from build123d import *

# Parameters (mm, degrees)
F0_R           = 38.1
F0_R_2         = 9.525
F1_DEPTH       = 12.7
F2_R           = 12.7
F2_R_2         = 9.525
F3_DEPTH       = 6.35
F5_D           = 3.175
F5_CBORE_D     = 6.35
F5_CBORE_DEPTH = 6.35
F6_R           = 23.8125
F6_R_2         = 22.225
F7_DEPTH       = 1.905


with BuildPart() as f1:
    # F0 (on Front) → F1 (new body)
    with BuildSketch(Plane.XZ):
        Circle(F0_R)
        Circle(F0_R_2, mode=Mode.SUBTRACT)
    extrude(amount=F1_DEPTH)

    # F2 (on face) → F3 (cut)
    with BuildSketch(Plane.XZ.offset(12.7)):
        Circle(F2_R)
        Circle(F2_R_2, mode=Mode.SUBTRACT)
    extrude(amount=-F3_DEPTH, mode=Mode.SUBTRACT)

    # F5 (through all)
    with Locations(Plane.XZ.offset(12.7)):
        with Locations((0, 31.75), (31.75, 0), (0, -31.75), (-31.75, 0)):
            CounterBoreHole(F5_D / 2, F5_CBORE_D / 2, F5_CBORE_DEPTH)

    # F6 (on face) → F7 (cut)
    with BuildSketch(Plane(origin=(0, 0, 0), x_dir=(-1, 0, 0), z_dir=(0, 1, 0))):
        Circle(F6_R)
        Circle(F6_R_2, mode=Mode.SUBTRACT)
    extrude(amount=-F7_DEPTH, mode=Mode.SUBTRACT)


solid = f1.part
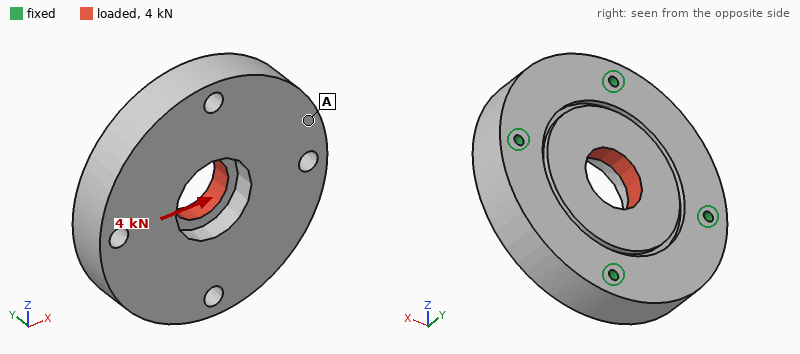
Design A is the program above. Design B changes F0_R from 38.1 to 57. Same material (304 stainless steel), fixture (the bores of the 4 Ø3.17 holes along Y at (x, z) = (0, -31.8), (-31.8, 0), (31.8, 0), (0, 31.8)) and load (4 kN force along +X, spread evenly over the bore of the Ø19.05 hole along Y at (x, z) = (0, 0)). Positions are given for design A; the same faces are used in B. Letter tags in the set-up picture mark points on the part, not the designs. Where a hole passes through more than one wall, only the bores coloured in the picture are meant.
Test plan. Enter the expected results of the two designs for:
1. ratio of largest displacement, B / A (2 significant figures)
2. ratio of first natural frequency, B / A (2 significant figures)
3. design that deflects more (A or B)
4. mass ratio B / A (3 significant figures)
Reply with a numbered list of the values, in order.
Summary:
1. 0.91
2. 0.44
3. A
4. 2.39
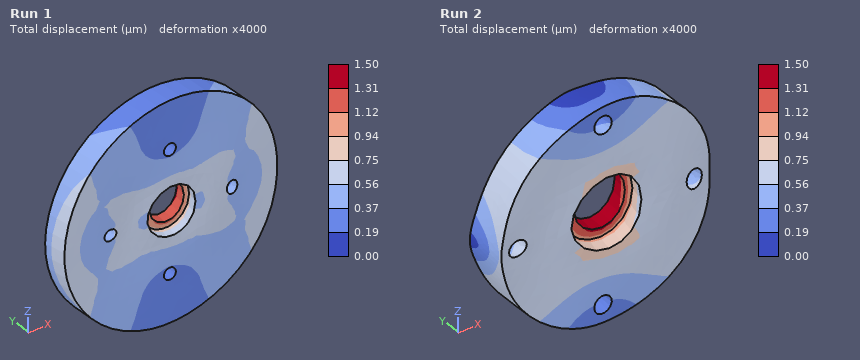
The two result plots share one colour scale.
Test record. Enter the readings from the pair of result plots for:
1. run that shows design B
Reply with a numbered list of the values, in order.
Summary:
1. Run 1
